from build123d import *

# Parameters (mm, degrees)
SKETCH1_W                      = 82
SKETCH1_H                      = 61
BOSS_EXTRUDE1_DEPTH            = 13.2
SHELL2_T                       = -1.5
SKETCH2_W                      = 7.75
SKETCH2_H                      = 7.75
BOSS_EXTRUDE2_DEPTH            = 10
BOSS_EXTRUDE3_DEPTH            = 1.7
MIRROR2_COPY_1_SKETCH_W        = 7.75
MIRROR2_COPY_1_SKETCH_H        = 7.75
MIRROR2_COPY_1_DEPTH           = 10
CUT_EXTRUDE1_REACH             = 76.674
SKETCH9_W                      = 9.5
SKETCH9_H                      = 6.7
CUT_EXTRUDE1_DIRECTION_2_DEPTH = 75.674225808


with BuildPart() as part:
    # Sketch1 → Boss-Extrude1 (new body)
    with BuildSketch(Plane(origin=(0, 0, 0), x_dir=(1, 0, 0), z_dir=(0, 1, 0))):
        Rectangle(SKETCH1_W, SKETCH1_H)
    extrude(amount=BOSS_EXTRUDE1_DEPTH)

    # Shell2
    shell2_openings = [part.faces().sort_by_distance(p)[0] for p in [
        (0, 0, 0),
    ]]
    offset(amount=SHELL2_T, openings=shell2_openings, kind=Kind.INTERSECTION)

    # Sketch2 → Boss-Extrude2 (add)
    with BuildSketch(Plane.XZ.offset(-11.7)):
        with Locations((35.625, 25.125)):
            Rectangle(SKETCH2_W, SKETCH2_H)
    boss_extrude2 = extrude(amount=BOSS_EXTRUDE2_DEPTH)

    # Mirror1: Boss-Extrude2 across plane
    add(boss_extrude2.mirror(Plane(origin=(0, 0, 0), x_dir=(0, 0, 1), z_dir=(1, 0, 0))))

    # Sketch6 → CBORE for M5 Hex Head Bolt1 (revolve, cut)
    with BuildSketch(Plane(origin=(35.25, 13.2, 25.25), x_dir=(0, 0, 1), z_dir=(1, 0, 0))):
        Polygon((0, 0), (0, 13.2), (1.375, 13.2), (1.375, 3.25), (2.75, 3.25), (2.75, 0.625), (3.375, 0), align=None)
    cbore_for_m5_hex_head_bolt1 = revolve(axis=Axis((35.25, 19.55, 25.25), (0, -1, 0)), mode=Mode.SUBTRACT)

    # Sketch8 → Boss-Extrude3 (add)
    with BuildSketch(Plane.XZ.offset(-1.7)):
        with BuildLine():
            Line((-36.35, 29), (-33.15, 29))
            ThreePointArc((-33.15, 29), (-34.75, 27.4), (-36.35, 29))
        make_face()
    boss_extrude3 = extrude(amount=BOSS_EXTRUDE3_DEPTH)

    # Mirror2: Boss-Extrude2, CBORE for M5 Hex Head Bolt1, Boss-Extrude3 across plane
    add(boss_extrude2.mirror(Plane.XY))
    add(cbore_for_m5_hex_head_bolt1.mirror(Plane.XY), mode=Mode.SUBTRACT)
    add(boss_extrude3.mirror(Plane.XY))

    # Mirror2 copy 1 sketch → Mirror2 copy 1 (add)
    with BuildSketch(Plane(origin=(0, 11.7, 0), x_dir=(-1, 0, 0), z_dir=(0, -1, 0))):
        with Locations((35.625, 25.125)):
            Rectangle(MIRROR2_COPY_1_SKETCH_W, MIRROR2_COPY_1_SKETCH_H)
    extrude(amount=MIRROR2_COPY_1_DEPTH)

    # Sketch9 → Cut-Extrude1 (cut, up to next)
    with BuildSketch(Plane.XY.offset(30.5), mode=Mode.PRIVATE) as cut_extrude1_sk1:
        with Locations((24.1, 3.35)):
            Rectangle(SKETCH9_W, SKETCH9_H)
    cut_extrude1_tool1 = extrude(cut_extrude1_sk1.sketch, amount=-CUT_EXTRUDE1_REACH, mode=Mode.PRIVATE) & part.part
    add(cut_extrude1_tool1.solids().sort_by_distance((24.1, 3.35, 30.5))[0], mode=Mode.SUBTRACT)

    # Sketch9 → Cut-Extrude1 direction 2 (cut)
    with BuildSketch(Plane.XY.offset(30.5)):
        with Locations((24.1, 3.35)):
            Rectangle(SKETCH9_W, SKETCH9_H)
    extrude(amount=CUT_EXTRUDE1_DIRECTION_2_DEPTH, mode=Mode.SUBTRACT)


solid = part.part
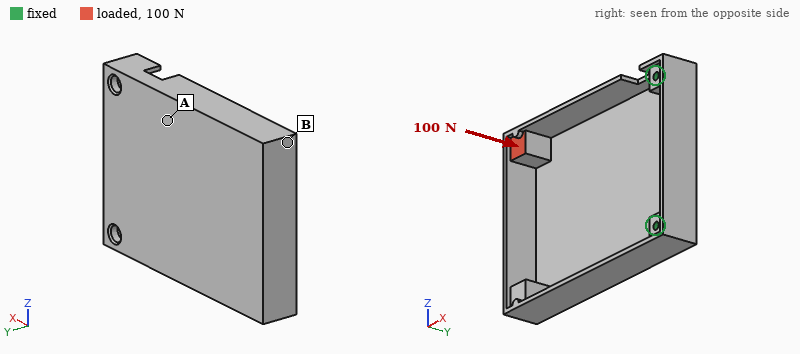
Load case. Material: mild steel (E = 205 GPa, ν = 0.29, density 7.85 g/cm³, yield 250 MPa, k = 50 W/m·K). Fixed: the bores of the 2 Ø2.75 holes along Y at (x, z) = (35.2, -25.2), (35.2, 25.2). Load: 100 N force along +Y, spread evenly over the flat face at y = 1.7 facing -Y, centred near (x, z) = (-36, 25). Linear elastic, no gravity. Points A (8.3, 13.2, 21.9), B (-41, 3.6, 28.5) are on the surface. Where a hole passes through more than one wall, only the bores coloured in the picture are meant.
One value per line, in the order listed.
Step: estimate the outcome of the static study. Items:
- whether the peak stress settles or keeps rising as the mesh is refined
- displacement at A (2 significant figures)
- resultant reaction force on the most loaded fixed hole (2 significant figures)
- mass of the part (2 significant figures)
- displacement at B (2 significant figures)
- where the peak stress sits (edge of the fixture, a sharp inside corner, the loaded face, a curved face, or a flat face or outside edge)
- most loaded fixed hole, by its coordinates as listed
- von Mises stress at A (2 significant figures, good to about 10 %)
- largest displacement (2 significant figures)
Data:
keeps rising
0.080 mm
110 N
110 g
0.38 mm
a sharp inside corner
(35.2, 25.2)
35 MPa
0.39 mm
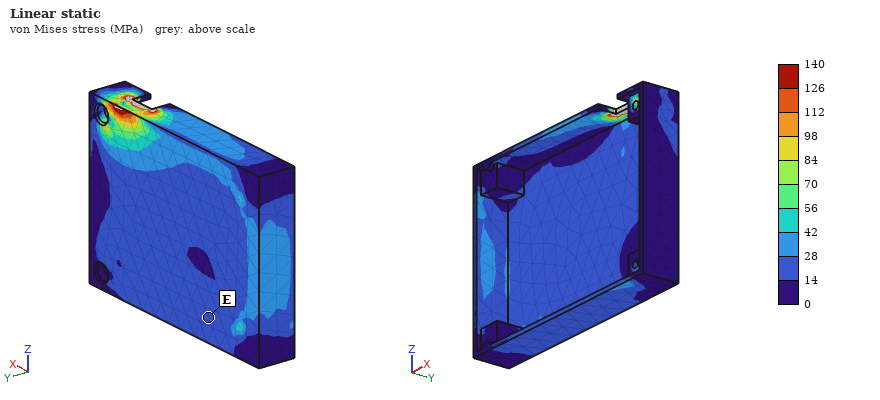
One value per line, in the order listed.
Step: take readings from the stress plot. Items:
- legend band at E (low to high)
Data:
14 to 28 MPa
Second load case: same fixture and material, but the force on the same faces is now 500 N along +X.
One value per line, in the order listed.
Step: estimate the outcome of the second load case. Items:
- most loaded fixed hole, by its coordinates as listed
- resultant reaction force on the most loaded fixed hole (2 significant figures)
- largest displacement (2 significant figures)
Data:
(35.2, 25.2)
460 N
0.34 mm
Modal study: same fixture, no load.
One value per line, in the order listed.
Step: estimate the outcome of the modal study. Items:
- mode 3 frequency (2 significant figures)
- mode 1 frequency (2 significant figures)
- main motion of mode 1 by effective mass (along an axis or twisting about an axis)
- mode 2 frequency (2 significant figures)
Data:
2300 Hz
600 Hz
along Y
1100 Hz
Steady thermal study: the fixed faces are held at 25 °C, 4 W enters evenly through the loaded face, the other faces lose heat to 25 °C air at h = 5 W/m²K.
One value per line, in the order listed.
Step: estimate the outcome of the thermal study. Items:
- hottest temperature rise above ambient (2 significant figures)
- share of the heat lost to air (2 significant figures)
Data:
58 K
38 %
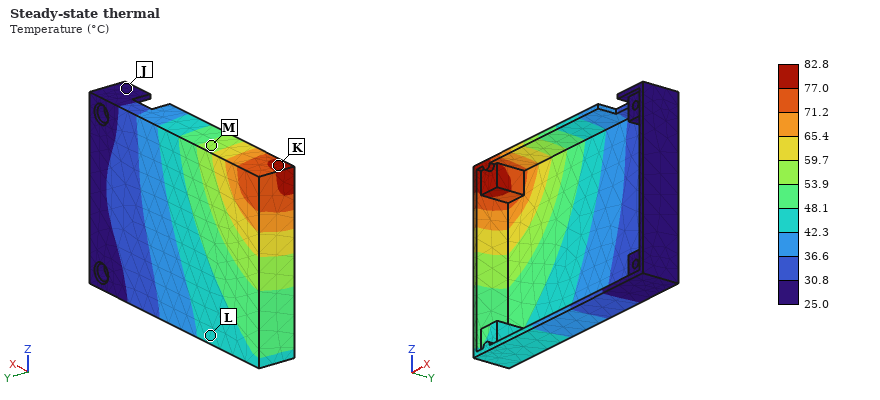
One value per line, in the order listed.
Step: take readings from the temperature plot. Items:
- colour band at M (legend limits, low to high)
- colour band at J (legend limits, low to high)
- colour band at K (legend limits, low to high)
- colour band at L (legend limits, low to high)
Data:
53.9 to 59.7 °C
25.0 to 30.8 °C
77.0 to 82.8 °C
42.3 to 48.1 °C
